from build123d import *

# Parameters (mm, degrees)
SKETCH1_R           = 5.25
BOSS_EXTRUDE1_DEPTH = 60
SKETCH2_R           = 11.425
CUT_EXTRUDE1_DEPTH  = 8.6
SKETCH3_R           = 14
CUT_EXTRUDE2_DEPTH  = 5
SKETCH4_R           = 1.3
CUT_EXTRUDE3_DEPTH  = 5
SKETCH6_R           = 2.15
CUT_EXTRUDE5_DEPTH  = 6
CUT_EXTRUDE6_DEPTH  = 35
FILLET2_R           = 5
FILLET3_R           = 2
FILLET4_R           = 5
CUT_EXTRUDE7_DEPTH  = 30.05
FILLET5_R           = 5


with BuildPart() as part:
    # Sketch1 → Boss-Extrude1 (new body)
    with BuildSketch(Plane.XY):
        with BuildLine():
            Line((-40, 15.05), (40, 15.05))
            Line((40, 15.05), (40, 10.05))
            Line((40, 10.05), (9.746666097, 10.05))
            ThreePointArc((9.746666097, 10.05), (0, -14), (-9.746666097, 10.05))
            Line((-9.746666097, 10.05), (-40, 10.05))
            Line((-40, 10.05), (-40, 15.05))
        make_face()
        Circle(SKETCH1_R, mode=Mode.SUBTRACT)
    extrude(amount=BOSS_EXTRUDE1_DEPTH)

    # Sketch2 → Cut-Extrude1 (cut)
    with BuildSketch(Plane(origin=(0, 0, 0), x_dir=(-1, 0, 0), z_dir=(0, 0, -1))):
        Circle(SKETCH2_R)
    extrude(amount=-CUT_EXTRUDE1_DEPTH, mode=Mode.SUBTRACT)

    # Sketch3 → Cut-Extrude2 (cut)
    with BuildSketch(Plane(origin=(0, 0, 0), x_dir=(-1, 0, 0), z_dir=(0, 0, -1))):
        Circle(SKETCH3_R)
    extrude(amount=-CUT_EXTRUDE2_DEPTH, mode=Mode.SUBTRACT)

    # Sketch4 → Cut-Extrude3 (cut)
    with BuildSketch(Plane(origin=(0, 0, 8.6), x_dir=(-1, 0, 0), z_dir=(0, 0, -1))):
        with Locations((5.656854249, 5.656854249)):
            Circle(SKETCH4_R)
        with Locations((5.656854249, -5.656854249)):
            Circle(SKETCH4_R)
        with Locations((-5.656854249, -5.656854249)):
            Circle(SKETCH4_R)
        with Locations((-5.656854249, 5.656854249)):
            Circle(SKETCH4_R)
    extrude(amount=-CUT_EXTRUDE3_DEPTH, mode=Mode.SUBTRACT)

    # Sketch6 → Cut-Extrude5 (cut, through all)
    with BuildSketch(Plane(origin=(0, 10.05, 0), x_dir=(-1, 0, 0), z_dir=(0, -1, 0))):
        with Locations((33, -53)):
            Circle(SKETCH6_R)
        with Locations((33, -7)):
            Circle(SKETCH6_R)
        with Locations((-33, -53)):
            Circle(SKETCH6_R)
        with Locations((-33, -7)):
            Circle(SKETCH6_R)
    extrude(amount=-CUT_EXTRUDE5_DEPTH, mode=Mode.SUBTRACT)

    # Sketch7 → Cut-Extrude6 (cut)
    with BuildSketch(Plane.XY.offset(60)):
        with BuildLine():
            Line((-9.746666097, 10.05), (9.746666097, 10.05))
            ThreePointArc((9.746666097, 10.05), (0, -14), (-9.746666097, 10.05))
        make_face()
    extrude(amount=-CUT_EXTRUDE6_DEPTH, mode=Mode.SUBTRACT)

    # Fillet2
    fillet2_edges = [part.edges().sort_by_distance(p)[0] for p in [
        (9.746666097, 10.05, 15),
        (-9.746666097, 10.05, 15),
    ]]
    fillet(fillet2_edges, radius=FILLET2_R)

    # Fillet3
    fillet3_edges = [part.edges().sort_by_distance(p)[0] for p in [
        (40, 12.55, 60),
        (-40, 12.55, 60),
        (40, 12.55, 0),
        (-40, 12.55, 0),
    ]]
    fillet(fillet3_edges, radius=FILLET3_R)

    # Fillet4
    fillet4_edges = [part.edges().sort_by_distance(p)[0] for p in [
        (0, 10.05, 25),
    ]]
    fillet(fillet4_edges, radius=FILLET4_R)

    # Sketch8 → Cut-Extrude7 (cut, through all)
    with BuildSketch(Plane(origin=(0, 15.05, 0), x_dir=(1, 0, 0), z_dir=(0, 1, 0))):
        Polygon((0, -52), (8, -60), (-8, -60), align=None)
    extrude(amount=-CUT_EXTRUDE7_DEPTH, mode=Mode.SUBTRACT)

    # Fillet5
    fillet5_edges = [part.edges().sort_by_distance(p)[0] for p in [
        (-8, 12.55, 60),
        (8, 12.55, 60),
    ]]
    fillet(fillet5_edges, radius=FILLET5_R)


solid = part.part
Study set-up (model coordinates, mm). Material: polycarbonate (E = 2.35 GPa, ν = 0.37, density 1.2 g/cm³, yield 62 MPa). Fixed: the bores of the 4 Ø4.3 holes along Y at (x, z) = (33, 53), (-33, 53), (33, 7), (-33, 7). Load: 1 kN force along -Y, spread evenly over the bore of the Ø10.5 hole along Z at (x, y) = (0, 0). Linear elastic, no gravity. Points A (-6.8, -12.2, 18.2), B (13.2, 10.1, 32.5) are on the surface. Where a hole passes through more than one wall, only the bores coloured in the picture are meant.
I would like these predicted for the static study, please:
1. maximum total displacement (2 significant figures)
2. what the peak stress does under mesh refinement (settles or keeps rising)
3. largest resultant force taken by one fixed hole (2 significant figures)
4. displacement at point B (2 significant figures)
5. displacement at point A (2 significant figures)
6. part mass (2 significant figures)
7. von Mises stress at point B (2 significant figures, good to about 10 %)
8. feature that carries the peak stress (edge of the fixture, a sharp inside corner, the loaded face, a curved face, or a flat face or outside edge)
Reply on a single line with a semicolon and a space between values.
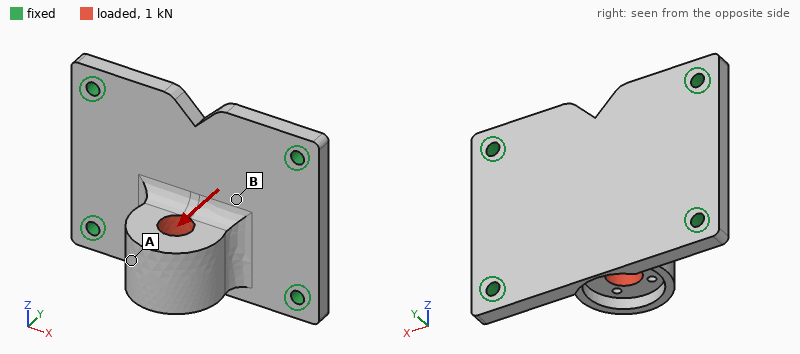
0.78 mm; keeps rising; 440 N; 0.57 mm; 0.67 mm; 38 g; 10 MPa; edge of the fixture
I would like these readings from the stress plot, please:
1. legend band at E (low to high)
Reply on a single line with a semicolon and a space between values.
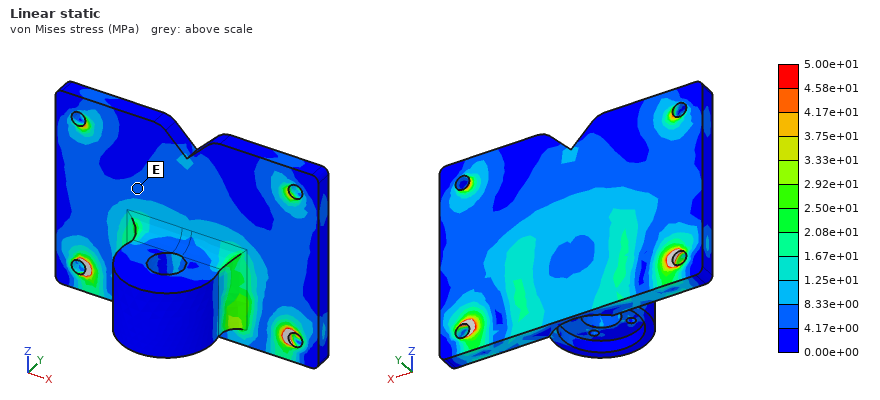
4.17e+00 to 8.33e+00 MPa
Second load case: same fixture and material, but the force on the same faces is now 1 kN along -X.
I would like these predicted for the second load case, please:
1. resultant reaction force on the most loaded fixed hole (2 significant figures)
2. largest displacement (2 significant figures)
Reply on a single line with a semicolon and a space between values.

410 N; 0.40 mm
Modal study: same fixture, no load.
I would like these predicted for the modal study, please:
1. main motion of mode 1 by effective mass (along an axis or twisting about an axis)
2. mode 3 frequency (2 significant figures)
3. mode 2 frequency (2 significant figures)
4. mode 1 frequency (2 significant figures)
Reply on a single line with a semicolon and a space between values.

along Y; 2200 Hz; 1500 Hz; 1300 Hz
